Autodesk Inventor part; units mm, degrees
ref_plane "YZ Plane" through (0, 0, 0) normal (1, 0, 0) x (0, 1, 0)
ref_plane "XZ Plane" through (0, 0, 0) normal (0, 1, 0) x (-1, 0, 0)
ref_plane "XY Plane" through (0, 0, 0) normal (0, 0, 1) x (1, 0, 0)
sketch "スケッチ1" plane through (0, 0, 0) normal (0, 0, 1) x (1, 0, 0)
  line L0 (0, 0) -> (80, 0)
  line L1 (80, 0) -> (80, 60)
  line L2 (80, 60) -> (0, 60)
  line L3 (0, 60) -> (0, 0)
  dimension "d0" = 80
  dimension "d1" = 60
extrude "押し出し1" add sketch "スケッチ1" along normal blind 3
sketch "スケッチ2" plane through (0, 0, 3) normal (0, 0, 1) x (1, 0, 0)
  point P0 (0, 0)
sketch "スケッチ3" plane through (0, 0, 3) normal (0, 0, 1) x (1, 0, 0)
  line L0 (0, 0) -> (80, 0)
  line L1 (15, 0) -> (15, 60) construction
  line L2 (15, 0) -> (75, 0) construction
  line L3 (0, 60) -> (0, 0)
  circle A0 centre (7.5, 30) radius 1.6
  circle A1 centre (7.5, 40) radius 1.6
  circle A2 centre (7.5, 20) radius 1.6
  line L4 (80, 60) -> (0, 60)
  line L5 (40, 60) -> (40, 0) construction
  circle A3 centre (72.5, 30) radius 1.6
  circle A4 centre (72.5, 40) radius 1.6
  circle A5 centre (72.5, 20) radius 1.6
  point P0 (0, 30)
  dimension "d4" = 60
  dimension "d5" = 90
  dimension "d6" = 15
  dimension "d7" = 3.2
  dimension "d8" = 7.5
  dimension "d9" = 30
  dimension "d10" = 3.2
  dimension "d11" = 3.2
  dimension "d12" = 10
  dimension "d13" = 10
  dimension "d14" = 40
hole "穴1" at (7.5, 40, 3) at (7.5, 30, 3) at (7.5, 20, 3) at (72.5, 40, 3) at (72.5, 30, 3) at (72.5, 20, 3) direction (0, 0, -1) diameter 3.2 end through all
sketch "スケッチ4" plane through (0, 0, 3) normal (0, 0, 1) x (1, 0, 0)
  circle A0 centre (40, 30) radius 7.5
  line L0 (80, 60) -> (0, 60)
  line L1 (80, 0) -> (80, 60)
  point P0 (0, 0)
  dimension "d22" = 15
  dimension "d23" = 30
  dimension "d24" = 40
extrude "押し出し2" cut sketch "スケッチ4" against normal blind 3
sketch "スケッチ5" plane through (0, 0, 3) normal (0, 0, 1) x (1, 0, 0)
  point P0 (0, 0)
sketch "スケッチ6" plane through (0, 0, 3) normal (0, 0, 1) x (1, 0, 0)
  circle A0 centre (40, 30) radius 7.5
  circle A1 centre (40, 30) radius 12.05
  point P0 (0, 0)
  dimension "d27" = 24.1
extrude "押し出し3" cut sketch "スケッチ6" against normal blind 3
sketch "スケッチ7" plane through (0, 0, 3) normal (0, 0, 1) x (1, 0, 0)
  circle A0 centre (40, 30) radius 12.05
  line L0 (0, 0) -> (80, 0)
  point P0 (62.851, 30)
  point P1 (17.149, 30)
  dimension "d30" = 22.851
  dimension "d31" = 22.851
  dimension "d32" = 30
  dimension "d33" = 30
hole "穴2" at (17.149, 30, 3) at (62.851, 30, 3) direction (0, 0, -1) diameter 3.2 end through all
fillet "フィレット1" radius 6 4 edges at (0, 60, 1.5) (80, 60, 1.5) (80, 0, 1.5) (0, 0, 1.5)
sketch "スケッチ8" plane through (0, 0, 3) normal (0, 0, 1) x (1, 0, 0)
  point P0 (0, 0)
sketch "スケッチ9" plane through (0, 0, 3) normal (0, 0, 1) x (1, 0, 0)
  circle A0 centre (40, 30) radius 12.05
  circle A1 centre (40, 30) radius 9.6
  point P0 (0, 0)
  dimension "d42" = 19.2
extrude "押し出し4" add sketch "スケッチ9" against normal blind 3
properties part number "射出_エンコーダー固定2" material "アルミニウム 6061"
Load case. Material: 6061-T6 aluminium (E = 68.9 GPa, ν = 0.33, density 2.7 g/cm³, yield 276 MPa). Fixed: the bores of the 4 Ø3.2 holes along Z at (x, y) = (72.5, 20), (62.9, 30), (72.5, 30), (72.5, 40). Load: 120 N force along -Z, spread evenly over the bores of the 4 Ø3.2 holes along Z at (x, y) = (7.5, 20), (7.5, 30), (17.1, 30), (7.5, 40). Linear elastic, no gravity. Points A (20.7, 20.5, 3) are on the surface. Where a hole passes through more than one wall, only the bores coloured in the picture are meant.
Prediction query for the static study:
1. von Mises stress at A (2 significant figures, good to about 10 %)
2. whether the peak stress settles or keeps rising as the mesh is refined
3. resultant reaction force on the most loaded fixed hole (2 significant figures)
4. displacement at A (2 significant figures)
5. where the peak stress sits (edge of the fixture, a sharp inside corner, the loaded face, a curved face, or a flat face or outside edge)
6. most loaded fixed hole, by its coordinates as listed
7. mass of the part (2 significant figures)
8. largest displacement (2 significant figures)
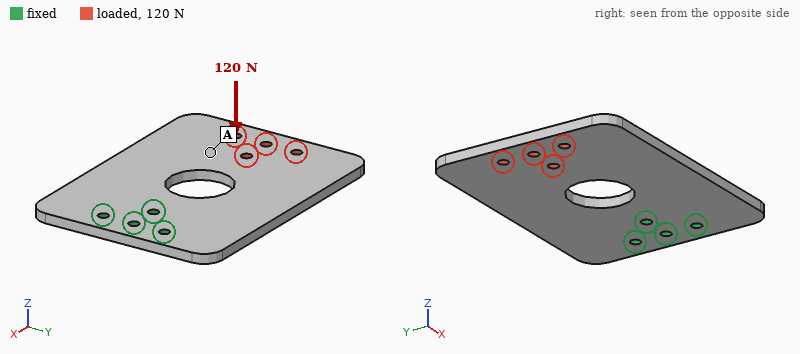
14 MPa
keeps rising
420 N
0.65 mm
edge of the fixture
(62.9, 30)
36 g
1.2 mm
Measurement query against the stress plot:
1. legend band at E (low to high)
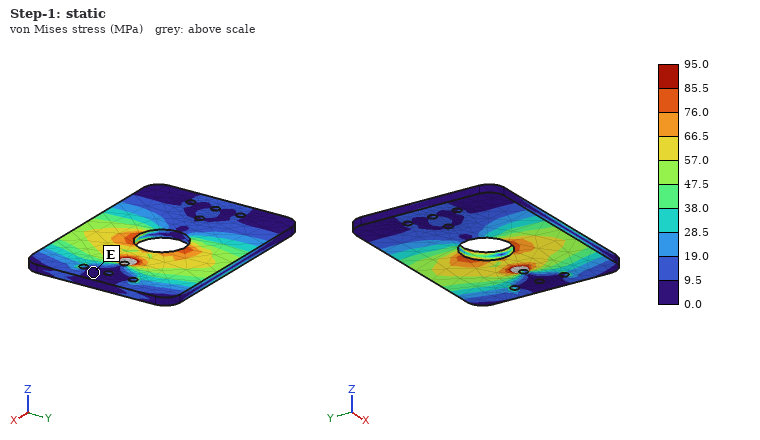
0.0 to 9.5 MPa
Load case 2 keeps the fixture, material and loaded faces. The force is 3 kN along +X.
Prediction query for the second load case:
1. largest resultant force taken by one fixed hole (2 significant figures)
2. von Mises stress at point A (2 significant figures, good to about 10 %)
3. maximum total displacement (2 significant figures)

1.1 kN
33 MPa
35 µm
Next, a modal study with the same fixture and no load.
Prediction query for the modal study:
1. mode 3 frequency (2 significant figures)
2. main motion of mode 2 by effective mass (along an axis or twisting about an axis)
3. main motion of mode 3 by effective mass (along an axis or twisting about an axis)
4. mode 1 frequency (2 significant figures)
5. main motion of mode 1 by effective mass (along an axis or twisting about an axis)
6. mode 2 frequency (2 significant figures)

2900 Hz
twisting about X
along Z
530 Hz
along Z
1100 Hz
